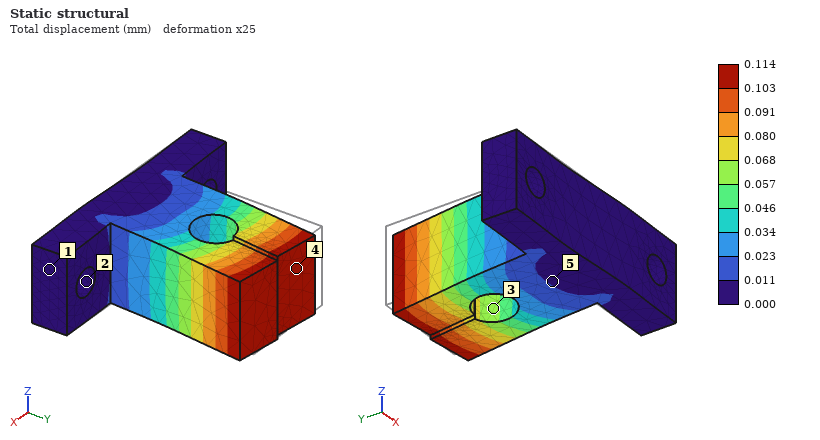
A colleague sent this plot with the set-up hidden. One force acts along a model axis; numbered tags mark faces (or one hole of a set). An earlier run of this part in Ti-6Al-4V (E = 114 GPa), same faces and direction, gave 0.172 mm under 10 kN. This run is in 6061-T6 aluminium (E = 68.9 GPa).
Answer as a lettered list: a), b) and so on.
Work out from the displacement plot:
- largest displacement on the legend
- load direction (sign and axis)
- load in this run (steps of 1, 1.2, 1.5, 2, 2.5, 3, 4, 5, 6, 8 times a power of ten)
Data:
a) 0.114 mm
b) +X
c) 4 kN
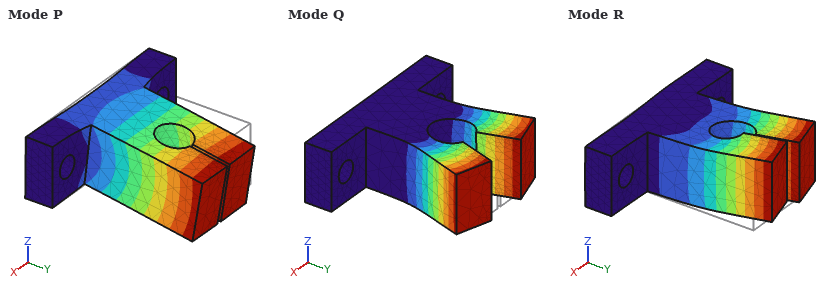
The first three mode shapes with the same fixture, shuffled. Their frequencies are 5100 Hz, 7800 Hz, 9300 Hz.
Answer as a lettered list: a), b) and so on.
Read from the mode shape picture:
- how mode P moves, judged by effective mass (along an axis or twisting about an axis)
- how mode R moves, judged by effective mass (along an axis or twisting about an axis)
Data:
a) along Z
b) along X
